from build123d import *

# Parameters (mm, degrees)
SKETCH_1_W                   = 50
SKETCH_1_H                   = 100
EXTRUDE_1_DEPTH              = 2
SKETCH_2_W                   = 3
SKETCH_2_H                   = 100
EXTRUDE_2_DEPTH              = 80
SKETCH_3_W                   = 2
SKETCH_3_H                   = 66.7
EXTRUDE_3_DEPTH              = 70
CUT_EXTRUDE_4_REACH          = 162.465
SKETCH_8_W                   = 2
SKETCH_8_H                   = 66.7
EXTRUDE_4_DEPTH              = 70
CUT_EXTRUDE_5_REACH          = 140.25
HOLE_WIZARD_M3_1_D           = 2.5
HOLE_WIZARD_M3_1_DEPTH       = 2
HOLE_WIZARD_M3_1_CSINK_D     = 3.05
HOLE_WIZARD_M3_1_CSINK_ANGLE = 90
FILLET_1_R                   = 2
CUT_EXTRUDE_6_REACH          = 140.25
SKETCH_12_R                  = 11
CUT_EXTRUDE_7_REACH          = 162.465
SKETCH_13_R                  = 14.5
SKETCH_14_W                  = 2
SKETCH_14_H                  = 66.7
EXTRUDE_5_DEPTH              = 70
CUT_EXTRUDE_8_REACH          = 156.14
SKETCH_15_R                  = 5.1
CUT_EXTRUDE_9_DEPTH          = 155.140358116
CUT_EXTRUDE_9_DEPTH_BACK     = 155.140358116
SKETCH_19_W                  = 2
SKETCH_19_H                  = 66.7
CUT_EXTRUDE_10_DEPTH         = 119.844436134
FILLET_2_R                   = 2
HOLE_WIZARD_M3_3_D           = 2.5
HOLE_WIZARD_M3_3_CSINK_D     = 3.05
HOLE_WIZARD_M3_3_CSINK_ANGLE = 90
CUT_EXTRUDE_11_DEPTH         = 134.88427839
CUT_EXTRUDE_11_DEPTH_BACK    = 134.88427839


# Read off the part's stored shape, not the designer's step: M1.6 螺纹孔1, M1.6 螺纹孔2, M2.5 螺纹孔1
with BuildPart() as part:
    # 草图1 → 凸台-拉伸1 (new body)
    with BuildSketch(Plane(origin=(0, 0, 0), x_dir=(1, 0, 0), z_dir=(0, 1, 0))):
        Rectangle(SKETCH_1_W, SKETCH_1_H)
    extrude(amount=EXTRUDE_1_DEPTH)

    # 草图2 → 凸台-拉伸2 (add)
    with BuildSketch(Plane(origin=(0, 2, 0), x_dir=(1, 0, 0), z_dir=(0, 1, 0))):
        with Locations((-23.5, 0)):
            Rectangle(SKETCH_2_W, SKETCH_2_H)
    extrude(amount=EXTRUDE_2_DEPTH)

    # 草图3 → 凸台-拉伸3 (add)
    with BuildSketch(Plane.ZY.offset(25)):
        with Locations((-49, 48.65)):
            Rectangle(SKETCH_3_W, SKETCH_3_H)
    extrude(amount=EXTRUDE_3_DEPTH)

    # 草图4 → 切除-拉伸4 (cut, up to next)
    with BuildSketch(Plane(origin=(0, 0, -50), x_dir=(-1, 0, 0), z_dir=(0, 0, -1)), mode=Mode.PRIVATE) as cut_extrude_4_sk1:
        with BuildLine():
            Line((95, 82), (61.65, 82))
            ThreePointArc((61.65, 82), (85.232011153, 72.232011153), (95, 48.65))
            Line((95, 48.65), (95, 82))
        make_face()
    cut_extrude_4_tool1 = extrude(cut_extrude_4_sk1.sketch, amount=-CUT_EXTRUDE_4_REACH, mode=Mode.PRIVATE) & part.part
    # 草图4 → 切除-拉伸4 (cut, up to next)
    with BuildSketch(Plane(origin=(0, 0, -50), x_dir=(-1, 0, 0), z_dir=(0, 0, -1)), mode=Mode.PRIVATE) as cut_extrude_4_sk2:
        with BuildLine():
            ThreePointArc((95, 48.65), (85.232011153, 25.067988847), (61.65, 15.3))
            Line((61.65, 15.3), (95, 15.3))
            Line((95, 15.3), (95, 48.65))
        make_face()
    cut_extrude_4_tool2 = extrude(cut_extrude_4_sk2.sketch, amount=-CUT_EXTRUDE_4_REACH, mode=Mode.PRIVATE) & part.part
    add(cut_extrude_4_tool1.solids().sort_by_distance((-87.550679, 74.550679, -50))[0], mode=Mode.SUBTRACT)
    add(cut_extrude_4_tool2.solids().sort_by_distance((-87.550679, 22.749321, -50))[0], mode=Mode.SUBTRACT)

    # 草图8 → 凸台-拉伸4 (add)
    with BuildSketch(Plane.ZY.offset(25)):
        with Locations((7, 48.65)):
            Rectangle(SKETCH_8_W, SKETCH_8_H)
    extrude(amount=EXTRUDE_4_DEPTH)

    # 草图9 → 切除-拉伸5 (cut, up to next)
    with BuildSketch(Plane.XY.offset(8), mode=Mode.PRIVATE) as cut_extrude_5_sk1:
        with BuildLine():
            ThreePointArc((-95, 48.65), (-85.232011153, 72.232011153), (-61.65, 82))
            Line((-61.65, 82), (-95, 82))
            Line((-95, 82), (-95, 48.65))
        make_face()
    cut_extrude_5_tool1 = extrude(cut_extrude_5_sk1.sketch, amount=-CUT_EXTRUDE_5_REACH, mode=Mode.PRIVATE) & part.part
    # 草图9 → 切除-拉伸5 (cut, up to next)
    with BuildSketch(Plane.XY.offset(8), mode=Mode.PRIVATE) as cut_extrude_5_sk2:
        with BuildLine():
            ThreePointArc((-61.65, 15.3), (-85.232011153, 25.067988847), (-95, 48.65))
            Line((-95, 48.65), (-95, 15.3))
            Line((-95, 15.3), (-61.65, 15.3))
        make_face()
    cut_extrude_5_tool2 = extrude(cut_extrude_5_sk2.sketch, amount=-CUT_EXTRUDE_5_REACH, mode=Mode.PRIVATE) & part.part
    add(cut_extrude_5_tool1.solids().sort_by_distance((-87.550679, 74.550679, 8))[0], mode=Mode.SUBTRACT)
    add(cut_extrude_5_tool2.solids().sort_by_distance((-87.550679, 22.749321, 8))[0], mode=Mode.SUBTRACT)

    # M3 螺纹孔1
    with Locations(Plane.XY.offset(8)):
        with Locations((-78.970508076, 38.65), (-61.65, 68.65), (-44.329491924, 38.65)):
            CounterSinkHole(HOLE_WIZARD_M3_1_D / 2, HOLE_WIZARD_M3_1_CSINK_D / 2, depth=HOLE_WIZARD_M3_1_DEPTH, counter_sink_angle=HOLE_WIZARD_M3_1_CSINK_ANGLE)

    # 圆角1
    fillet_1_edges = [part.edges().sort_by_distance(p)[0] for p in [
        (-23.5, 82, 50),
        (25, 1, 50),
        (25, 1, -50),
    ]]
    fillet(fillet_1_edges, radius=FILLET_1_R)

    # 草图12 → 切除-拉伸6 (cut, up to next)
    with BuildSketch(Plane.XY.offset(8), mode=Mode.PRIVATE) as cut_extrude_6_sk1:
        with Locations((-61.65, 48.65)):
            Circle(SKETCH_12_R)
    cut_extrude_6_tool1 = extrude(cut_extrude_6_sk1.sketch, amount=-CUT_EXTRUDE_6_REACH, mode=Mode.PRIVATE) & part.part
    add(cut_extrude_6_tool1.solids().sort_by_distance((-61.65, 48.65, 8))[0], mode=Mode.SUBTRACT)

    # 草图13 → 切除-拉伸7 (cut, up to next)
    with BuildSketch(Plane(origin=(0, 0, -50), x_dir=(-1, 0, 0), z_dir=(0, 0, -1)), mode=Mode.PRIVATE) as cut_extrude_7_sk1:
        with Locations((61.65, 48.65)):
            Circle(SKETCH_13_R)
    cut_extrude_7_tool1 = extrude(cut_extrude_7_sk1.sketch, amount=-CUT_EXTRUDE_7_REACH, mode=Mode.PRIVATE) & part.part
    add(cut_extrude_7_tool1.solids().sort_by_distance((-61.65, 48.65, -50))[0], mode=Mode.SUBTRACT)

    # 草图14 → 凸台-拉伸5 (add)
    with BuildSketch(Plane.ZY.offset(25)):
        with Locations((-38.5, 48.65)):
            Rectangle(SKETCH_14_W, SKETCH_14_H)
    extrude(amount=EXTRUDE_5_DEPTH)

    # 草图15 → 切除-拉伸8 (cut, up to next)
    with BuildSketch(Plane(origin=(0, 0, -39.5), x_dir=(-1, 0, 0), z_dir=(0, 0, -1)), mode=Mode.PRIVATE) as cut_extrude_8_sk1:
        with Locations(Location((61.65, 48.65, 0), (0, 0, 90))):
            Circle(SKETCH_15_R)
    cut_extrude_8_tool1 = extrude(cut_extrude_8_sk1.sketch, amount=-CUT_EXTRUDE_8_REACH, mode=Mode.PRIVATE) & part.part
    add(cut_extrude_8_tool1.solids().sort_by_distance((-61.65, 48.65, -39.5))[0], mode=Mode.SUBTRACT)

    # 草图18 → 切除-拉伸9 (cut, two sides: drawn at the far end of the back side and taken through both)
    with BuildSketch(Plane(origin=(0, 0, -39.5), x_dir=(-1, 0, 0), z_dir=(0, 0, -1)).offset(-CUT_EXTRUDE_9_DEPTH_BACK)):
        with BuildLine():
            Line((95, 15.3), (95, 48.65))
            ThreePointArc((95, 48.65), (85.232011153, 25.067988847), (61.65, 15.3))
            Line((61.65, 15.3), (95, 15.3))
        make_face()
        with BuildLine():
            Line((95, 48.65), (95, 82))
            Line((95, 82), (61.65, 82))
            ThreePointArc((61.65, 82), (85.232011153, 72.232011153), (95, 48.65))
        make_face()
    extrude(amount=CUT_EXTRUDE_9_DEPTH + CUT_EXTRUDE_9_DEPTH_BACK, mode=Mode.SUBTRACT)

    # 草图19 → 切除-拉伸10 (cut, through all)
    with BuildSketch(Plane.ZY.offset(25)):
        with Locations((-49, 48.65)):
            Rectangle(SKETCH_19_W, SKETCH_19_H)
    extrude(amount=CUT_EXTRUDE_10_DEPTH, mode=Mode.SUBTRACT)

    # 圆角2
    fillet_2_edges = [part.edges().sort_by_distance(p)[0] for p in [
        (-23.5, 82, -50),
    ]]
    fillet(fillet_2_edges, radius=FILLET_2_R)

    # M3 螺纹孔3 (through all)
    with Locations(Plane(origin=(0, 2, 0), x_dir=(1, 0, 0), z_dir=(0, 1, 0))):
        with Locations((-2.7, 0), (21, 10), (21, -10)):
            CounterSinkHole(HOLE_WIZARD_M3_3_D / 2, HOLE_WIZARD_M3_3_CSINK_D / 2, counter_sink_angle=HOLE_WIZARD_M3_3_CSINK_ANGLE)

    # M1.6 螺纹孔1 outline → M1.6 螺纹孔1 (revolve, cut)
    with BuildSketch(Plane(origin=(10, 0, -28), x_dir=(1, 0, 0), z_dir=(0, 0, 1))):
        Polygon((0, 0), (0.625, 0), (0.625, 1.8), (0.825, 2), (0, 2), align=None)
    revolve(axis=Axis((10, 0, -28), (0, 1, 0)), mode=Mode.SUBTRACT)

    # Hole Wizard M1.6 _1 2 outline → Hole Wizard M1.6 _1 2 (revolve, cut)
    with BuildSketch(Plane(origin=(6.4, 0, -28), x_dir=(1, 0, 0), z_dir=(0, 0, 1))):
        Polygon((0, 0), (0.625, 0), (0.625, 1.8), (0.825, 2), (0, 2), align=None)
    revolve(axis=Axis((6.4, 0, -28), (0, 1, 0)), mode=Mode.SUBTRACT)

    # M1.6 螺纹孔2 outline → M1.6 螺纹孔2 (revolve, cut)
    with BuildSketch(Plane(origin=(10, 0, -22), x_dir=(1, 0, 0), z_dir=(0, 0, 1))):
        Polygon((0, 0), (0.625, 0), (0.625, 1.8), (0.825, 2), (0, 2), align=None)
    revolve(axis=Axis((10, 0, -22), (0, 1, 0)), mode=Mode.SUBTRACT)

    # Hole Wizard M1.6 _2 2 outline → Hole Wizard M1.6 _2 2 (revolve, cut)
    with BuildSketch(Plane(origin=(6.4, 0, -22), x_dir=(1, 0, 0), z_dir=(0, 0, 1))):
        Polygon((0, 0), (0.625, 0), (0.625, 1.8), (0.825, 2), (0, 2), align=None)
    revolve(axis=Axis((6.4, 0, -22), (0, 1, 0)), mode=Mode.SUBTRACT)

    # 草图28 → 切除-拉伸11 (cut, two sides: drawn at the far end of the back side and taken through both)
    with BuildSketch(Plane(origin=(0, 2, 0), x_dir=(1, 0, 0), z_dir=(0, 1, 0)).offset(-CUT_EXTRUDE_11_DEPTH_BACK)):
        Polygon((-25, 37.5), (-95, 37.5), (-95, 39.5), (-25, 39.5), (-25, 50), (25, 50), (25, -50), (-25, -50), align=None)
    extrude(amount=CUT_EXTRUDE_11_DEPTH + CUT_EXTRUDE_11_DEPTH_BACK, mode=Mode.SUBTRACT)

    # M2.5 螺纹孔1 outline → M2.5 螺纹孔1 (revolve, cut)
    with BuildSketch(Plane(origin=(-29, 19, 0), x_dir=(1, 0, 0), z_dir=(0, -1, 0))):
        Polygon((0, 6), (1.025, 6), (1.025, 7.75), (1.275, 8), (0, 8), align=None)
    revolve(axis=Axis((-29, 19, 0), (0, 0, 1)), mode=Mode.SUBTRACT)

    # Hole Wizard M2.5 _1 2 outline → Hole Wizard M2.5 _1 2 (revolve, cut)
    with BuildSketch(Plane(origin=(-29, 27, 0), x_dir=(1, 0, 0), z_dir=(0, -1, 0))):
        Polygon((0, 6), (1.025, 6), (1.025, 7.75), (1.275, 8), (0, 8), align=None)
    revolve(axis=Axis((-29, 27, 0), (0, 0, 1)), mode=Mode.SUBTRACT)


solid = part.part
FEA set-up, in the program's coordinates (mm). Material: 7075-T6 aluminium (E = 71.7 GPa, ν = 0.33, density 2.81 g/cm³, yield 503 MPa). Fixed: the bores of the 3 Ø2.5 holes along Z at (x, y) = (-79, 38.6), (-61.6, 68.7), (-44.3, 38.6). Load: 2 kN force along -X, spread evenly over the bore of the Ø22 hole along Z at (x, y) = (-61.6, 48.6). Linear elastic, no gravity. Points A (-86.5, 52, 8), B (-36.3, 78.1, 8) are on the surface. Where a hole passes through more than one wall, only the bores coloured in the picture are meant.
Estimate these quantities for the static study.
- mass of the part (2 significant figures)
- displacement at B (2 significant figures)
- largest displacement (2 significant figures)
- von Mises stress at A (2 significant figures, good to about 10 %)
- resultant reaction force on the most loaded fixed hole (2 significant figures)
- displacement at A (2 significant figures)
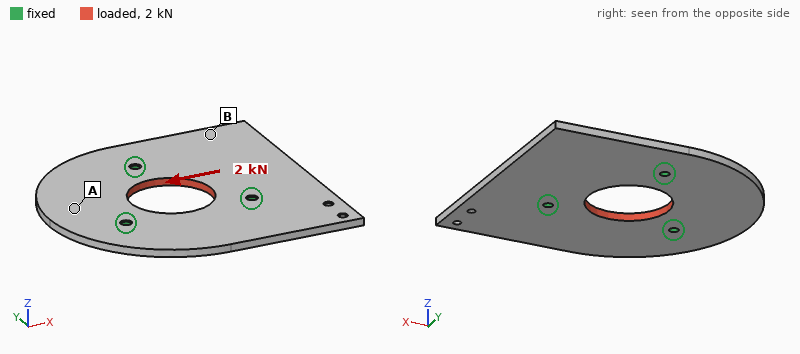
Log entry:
21 g
3.2 µm
6.7 µm
8.1 MPa
720 N
4.3 µm
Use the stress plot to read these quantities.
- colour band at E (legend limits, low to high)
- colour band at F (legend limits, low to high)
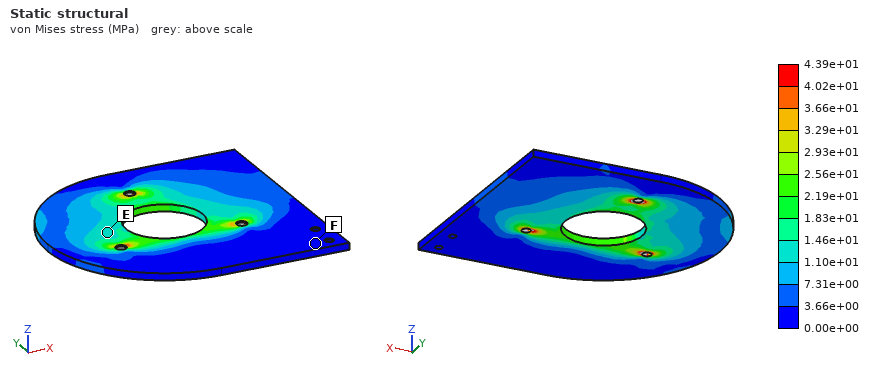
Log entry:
1.10e+01 to 1.46e+01 MPa
0.00e+00 to 3.66e+00 MPa
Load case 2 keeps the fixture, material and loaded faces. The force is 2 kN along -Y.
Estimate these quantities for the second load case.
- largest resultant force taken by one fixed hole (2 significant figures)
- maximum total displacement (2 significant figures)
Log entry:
700 N
7.3 µm
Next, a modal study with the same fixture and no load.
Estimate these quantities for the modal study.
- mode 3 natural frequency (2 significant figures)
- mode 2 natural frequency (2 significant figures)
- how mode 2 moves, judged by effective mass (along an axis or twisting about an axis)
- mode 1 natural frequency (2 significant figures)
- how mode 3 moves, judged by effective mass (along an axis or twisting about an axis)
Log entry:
3000 Hz
2500 Hz
along Z
1600 Hz
along Z
